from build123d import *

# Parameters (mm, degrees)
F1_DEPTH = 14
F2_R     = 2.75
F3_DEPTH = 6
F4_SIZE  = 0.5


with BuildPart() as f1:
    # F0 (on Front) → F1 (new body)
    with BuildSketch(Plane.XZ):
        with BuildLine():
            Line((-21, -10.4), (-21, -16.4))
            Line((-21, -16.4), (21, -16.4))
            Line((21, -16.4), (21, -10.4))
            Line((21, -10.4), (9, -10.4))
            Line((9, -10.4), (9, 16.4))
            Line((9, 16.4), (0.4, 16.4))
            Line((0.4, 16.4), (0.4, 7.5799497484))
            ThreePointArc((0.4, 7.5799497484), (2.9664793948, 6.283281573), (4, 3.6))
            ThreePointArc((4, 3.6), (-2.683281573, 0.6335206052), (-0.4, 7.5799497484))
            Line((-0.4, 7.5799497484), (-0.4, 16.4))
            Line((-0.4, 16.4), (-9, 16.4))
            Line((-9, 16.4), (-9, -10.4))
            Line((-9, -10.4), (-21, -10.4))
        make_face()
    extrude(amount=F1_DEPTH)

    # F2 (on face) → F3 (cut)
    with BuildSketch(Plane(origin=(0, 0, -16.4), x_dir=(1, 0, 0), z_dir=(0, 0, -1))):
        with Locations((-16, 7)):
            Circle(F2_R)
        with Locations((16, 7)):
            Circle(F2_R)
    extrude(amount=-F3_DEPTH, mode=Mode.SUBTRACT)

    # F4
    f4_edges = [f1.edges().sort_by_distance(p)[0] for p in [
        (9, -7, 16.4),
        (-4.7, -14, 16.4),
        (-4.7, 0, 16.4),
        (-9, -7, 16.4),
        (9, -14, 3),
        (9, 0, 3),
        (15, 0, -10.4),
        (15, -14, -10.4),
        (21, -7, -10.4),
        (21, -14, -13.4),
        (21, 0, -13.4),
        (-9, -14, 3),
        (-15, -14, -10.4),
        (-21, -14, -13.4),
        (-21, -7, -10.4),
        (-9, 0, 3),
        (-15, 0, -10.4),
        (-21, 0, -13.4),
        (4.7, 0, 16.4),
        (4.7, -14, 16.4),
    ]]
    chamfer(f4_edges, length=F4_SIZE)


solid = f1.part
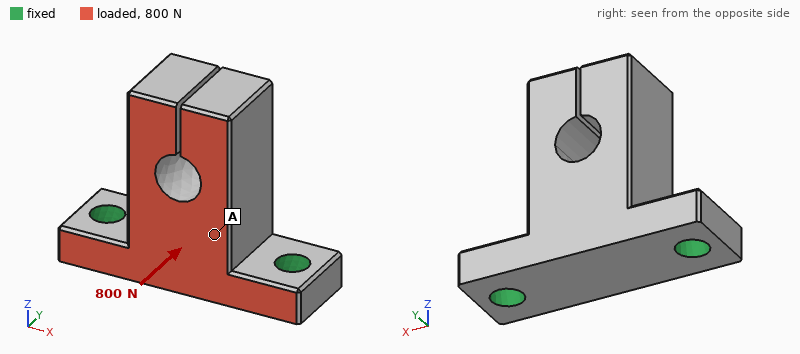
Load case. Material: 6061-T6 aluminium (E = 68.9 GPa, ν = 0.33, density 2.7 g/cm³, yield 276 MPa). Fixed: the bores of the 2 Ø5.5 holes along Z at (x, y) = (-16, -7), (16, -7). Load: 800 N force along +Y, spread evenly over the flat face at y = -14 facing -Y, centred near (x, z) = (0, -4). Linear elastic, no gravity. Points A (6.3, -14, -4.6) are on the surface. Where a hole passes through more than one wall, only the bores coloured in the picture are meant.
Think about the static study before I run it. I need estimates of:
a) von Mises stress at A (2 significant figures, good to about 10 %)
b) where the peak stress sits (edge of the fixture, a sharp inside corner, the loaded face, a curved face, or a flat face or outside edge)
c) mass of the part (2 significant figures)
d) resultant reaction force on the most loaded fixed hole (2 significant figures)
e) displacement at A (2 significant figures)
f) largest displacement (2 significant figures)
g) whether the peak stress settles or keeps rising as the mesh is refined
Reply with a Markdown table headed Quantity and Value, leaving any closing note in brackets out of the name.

| Quantity | Value |
|---|---|
| von Mises stress at A | 9.1 MPa |
| where the peak stress sits | edge of the fixture |
| mass of the part | 25 g |
| resultant reaction force on the most loaded fixed hole | 400 N |
| displacement at A | 17 µm |
| largest displacement | 48 µm |
| whether the peak stress settles or keeps rising as the mesh is refined | keeps rising |
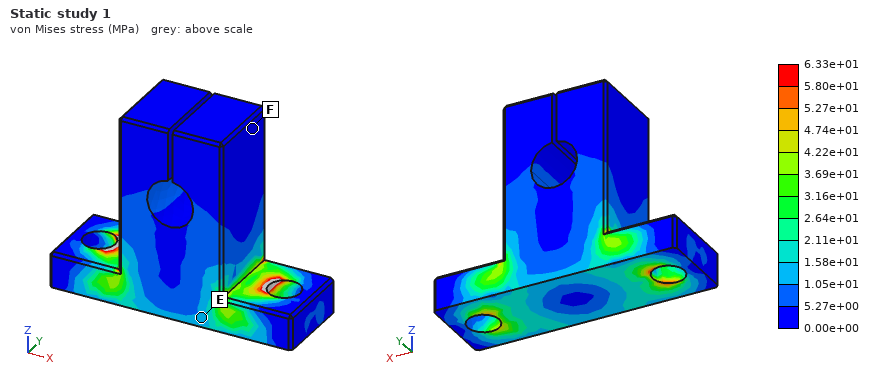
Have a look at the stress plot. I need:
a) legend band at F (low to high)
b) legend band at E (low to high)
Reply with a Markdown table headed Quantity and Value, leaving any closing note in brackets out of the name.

| Quantity | Value |
|---|---|
| legend band at F | 0.00e+00 to 5.27e+00 MPa |
| legend band at E | 1.05e+01 to 1.58e+01 MPa |
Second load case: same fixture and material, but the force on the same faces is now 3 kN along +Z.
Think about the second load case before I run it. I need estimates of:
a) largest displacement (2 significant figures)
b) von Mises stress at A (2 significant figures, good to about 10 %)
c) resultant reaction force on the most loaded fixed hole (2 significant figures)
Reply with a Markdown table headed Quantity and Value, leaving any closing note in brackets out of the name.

| Quantity | Value |
|---|---|
| largest displacement | 0.11 mm |
| von Mises stress at A | 32 MPa |
| resultant reaction force on the most loaded fixed hole | 1.6 kN |
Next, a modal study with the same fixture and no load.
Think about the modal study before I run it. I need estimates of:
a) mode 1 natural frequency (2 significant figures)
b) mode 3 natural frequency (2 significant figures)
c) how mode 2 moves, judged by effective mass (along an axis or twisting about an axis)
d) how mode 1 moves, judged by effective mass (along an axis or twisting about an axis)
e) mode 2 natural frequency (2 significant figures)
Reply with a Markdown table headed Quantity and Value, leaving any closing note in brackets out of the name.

| Quantity | Value |
|---|---|
| mode 1 natural frequency | 4900 Hz |
| mode 3 natural frequency | 9500 Hz |
| how mode 2 moves, judged by effective mass | along X |
| how mode 1 moves, judged by effective mass | along Y |
| mode 2 natural frequency | 7800 Hz |
